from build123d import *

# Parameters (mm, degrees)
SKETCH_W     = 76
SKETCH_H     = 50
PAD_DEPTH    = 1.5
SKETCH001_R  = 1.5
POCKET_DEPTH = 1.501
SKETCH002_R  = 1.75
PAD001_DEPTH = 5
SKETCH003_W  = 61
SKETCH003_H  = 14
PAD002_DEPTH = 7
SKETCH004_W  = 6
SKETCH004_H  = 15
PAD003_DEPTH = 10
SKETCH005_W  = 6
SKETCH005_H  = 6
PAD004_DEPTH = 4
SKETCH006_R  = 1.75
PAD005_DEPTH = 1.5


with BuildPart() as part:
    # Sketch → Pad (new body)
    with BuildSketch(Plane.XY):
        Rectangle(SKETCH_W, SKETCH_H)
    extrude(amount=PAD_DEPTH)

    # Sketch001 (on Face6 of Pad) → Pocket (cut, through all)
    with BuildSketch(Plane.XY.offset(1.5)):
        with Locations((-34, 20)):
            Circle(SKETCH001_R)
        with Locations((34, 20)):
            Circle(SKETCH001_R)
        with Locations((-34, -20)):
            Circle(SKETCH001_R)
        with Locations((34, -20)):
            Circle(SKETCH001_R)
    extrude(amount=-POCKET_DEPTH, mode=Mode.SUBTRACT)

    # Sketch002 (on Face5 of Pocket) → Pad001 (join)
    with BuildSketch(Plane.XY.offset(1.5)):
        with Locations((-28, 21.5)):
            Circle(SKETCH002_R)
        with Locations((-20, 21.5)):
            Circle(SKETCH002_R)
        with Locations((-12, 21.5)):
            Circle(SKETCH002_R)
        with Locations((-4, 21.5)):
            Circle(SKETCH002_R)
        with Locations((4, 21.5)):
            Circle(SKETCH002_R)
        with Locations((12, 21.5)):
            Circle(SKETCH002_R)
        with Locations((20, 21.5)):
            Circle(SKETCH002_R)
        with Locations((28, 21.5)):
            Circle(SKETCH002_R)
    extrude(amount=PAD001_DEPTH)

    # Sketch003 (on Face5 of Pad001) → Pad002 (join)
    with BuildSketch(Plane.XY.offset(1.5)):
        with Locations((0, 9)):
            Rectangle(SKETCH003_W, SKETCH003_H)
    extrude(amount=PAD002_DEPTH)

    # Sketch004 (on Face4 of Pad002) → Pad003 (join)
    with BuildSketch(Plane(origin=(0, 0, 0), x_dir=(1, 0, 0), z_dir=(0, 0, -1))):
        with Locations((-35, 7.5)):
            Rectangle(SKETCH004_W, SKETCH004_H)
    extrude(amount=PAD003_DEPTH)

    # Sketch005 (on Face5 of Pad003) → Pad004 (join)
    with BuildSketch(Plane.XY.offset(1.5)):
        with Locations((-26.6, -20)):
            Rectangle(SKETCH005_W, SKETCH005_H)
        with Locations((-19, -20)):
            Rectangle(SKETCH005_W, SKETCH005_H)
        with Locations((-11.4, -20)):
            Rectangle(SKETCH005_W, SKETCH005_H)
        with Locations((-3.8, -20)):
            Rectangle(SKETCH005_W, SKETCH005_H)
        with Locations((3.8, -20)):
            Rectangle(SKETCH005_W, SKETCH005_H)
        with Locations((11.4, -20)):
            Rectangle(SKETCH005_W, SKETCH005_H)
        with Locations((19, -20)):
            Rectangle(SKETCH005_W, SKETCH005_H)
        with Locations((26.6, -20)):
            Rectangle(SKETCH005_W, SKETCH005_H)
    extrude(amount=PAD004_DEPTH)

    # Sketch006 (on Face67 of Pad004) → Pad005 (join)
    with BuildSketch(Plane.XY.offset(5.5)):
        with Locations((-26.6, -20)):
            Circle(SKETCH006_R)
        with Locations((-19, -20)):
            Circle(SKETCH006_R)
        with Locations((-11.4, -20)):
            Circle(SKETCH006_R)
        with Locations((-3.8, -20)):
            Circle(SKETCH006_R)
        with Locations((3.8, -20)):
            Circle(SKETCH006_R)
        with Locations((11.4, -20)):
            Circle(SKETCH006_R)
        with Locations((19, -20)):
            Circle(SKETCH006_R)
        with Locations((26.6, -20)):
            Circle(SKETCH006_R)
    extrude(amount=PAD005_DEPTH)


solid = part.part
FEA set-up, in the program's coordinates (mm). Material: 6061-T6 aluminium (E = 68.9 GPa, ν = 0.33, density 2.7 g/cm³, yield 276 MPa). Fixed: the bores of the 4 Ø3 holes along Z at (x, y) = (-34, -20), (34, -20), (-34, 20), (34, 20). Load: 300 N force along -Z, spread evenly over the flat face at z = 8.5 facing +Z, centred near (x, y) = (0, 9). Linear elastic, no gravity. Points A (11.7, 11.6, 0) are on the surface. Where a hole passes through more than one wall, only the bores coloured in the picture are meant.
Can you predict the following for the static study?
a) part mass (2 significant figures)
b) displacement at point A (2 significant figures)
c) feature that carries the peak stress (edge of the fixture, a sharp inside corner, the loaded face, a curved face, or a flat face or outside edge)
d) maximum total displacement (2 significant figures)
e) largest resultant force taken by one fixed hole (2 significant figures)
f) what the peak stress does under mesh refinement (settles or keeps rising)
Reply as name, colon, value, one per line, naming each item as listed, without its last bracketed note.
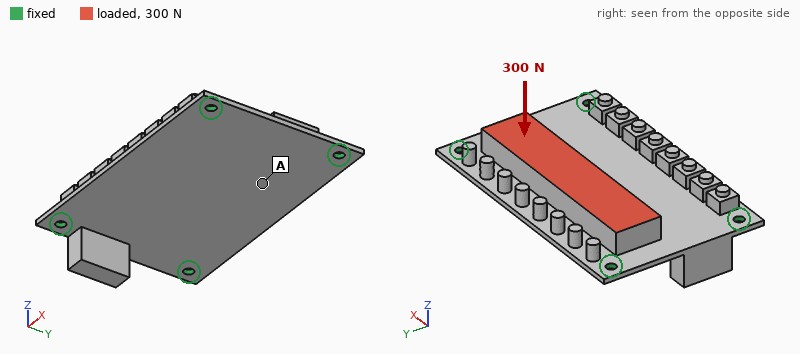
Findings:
part mass: 38 g
displacement at point A: 37 µm
feature that carries the peak stress: edge of the fixture
maximum total displacement: 67 µm
largest resultant force taken by one fixed hole: 170 N
what the peak stress does under mesh refinement: keeps rising
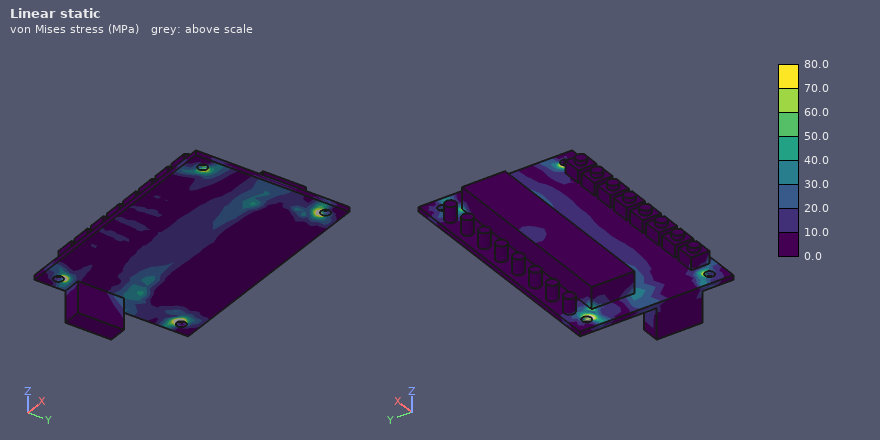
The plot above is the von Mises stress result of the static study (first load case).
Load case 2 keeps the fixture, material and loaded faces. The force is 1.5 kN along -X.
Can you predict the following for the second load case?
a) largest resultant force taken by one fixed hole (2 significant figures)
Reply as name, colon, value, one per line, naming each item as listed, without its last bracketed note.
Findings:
largest resultant force taken by one fixed hole: 580 N
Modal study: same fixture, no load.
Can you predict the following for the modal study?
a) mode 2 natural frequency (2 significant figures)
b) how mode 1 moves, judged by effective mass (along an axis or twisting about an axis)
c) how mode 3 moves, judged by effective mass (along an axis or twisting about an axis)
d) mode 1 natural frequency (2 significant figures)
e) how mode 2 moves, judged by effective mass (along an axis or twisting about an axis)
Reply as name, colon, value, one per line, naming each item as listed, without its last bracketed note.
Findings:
mode 2 natural frequency: 3100 Hz
how mode 1 moves, judged by effective mass: along Z
how mode 3 moves, judged by effective mass: twisting about Y
mode 1 natural frequency: 1900 Hz
how mode 2 moves, judged by effective mass: along Z
